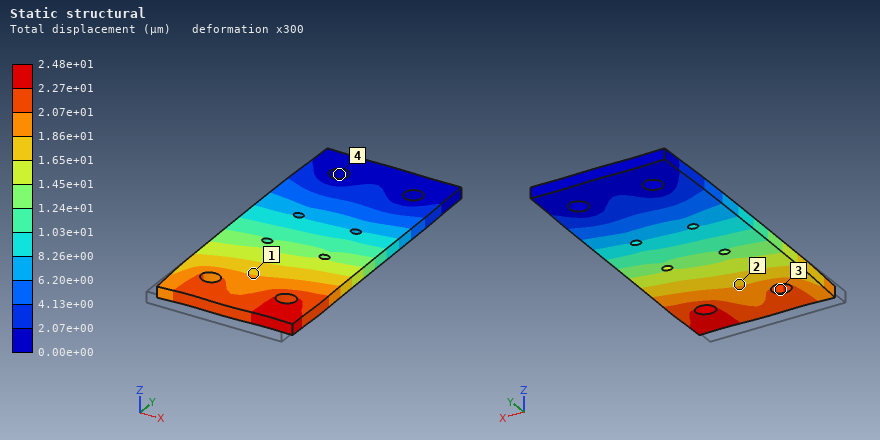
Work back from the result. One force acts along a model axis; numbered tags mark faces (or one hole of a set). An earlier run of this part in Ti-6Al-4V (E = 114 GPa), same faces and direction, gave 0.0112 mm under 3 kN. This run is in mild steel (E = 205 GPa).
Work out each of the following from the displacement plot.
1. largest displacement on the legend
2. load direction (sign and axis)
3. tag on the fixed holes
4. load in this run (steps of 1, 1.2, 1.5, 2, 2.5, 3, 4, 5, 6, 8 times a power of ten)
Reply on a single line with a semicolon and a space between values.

2.48e+01 µm; +Y; 4; 12 kN
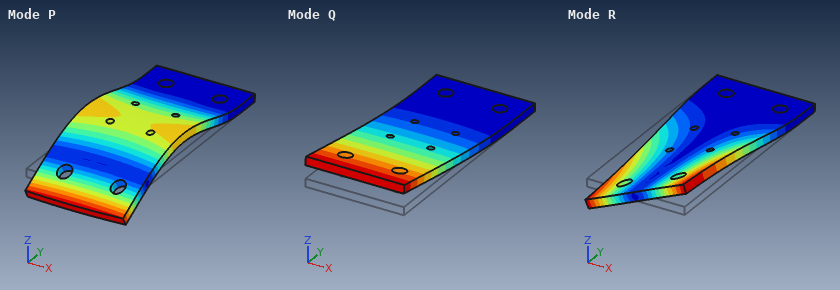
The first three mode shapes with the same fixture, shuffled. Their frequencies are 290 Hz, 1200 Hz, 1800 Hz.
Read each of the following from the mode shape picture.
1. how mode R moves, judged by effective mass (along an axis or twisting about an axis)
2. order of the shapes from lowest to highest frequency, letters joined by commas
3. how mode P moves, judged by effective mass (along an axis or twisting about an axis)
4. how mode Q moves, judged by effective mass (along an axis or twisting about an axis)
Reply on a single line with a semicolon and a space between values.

twisting about Y; Q, R, P; along Z; along Z
